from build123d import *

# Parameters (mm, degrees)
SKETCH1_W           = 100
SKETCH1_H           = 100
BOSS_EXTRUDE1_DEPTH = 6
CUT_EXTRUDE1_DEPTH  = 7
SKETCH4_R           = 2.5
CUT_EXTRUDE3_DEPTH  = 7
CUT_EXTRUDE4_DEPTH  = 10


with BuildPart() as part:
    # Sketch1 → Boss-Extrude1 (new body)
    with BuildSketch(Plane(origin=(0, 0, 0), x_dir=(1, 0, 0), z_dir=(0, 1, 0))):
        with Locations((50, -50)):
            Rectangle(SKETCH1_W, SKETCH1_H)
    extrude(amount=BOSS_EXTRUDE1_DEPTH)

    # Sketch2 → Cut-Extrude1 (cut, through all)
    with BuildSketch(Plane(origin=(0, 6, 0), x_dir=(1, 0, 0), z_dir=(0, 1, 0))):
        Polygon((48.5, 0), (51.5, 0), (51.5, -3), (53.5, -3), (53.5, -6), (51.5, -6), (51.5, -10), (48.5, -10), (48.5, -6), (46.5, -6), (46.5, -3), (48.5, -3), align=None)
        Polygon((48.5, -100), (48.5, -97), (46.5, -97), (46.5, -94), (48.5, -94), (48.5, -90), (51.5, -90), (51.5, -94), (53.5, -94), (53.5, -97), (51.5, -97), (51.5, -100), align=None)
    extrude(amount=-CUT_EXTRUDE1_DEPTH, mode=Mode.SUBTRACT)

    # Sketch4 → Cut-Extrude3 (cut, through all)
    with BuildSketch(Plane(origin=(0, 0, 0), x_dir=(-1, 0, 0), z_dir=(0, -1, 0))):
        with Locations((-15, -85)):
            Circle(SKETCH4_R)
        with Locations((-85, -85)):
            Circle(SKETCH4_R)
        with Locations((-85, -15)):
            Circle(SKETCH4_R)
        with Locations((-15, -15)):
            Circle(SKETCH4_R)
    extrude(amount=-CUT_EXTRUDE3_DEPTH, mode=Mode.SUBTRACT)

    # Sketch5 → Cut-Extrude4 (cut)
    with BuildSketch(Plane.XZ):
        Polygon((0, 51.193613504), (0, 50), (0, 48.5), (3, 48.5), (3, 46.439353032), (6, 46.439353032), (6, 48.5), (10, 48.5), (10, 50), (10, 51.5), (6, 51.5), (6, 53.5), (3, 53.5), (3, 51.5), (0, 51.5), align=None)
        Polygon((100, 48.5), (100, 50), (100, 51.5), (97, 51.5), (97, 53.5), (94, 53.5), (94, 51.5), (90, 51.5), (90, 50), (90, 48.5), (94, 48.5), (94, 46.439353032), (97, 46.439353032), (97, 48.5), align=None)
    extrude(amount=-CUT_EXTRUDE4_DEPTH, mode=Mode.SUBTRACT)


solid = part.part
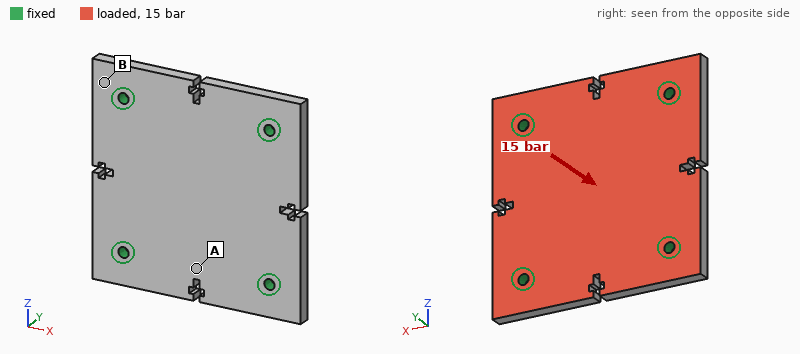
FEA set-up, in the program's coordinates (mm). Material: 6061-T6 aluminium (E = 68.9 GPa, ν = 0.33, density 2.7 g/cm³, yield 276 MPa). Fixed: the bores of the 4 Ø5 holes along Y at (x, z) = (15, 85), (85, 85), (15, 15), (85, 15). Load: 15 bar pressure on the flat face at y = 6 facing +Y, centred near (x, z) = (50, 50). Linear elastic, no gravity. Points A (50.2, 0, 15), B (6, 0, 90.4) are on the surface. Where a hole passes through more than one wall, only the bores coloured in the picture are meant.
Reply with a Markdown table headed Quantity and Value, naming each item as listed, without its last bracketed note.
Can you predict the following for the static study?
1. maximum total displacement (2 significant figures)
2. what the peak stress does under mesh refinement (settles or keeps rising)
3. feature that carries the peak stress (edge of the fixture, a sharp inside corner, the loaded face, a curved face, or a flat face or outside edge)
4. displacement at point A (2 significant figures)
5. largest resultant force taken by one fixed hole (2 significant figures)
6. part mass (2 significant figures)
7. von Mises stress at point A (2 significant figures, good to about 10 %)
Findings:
| Quantity | Value |
|---|---|
| maximum total displacement | 0.20 mm |
| what the peak stress does under mesh refinement | keeps rising |
| feature that carries the peak stress | edge of the fixture |
| displacement at point A | 0.12 mm |
| largest resultant force taken by one fixed hole | 3.7 kN |
| part mass | 160 g |
| von Mises stress at point A | 76 MPa |
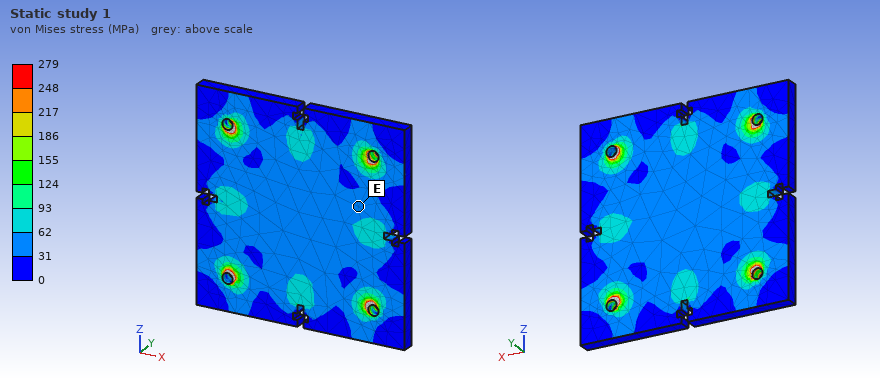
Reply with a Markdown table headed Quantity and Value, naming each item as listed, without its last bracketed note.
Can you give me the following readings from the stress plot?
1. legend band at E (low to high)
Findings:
| Quantity | Value |
|---|---|
| legend band at E | 31 to 62 MPa |
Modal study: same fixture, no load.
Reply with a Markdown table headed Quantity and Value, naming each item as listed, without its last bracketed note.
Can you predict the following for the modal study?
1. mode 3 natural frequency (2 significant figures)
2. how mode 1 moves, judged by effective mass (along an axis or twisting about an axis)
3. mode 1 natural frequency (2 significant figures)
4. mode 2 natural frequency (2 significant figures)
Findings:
| Quantity | Value |
|---|---|
| mode 3 natural frequency | 6000 Hz |
| how mode 1 moves, judged by effective mass | along Y |
| mode 1 natural frequency | 4200 Hz |
| mode 2 natural frequency | 5900 Hz |
